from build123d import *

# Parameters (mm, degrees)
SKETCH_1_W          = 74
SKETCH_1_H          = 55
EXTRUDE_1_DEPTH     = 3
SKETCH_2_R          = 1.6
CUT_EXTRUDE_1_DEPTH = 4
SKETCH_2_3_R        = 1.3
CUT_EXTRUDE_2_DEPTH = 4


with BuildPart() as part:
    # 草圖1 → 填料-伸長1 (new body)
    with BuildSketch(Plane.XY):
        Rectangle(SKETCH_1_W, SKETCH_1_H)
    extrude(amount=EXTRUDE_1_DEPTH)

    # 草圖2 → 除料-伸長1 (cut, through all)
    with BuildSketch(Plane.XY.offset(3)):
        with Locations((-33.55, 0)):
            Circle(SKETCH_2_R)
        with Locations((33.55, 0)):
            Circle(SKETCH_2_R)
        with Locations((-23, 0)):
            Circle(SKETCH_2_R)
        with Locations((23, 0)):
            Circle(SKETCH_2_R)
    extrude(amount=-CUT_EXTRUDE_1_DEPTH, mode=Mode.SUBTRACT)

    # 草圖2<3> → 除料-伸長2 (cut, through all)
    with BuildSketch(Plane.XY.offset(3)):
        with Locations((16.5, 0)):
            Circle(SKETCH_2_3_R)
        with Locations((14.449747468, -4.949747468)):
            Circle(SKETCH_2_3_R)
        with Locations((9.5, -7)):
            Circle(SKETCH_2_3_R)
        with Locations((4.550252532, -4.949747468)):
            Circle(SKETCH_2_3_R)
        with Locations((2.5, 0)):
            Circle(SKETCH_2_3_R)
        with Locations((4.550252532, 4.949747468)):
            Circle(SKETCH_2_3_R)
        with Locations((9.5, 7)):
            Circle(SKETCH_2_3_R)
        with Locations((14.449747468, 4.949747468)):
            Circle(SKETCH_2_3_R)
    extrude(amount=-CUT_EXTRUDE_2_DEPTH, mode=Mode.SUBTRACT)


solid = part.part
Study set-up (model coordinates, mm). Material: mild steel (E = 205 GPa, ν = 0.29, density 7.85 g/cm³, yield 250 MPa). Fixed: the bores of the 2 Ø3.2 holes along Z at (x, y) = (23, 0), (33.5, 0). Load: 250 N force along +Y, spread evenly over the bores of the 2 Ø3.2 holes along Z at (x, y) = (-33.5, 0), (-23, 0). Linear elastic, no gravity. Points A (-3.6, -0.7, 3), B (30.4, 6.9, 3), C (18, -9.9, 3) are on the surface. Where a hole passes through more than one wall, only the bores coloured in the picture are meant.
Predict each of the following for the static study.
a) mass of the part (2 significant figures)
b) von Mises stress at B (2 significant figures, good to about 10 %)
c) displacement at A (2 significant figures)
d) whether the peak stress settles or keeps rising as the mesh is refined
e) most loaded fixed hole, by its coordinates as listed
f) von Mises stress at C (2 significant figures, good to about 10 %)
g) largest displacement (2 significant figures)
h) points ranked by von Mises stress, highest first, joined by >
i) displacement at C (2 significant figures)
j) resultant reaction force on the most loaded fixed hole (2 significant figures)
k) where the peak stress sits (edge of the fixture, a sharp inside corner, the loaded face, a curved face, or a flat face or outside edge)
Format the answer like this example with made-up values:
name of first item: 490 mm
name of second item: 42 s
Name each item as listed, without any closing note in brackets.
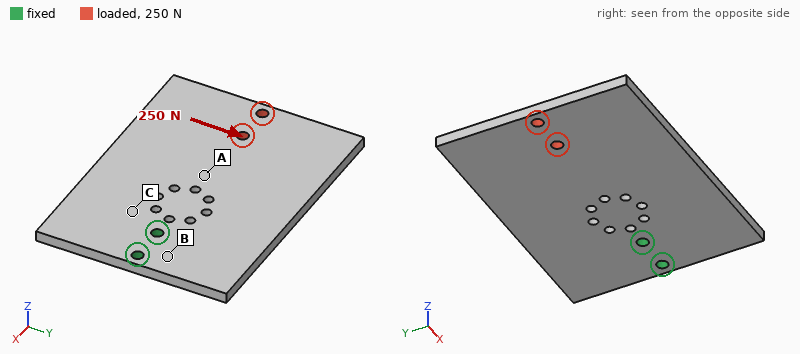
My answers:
mass of the part: 94 g
von Mises stress at B: 19 MPa
displacement at A: 7.9 µm
whether the peak stress settles or keeps rising as the mesh is refined: keeps rising
most loaded fixed hole, by its coordinates as listed: (23, 0)
von Mises stress at C: 10 MPa
largest displacement: 19 µm
points ranked by von Mises stress, highest first, joined by >: B > C > A
displacement at C: 3.0 µm
resultant reaction force on the most loaded fixed hole: 1.2 kN
where the peak stress sits: edge of the fixture
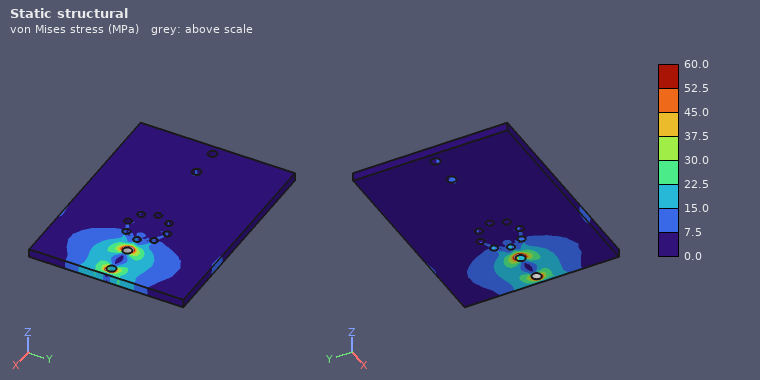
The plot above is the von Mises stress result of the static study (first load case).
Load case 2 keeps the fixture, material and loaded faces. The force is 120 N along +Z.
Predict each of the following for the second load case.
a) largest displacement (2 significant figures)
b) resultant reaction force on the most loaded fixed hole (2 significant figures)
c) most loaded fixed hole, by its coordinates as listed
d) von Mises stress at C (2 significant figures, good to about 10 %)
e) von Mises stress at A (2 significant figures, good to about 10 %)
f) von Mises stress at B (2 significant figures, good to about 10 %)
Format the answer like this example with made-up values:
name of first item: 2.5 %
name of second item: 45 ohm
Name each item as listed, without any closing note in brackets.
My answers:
largest displacement: 0.36 mm
resultant reaction force on the most loaded fixed hole: 430 N
most loaded fixed hole, by its coordinates as listed: (23, 0)
von Mises stress at C: 73 MPa
von Mises stress at A: 29 MPa
von Mises stress at B: 33 MPa
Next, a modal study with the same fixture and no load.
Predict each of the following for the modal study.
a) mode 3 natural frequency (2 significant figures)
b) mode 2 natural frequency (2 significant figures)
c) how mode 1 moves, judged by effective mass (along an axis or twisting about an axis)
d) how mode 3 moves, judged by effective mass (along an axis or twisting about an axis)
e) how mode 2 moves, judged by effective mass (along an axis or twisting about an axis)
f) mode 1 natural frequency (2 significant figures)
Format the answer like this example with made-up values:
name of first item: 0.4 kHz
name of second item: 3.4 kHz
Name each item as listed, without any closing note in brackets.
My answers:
mode 3 natural frequency: 3000 Hz
mode 2 natural frequency: 1200 Hz
how mode 1 moves, judged by effective mass: along Z
how mode 3 moves, judged by effective mass: along Z
how mode 2 moves, judged by effective mass: twisting about X
mode 1 natural frequency: 590 Hz
